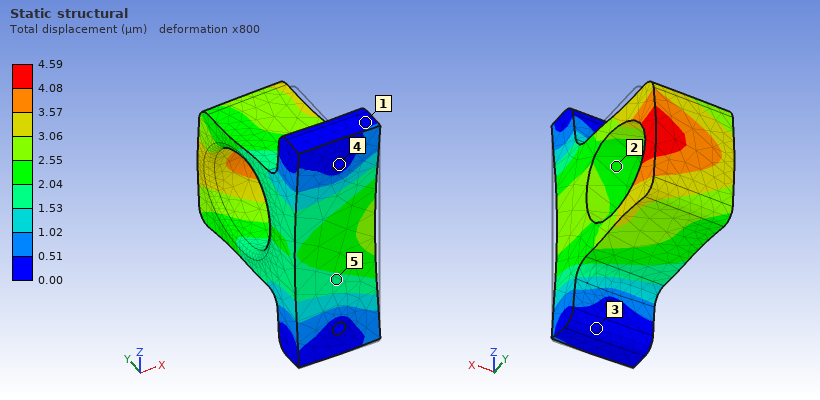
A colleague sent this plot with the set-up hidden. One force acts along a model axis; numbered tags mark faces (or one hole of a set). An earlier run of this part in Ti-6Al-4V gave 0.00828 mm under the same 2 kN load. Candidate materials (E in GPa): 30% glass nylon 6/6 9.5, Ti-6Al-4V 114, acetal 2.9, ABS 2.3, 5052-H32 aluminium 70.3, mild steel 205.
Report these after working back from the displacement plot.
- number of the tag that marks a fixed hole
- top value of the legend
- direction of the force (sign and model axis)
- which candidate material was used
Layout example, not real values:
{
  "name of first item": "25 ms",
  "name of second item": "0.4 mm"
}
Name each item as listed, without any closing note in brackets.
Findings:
{
  "number of the tag that marks a fixed hole": "4",
  "top value of the legend": "4.59 µm",
  "direction of the force": "+Y",
  "which candidate material was used": "mild steel"
}
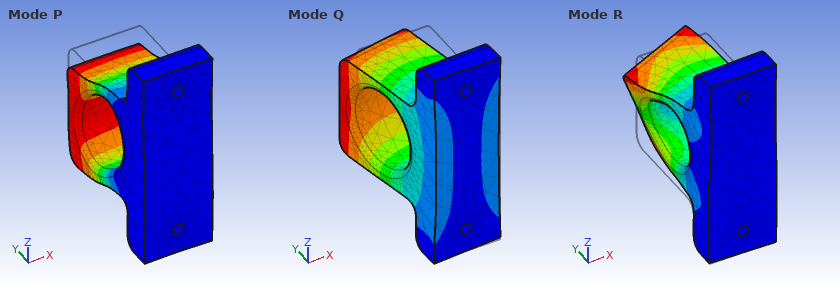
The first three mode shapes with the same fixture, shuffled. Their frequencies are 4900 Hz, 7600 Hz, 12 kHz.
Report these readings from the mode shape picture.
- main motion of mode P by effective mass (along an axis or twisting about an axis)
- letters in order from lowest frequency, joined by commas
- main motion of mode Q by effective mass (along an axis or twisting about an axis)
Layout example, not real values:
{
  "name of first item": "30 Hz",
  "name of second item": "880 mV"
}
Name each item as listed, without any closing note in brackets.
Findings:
{
  "main motion of mode P by effective mass": "along Z",
  "letters in order from lowest frequency, joined by commas": "Q, P, R",
  "main motion of mode Q by effective mass": "along X"
}
